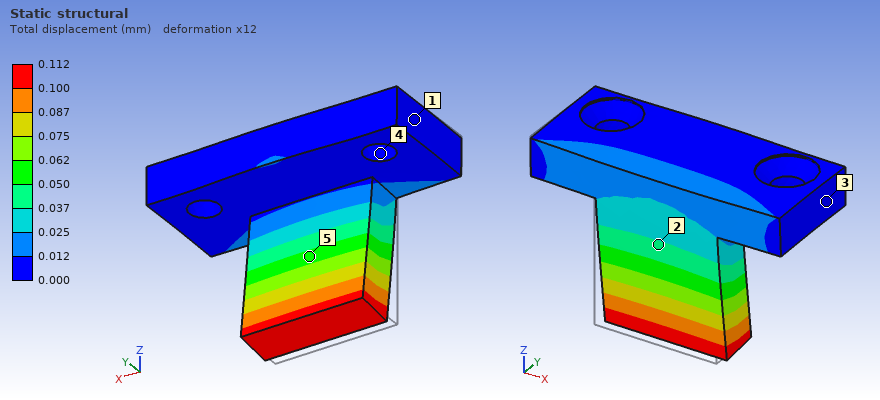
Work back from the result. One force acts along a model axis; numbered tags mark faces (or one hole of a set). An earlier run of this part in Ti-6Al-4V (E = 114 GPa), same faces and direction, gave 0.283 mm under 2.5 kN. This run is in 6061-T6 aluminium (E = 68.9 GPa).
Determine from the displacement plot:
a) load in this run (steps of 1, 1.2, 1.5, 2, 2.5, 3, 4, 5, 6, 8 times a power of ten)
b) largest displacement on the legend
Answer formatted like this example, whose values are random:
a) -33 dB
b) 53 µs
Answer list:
a) 600 N
b) 0.112 mm
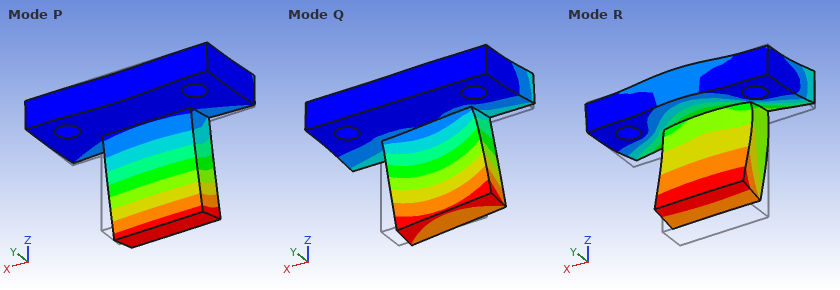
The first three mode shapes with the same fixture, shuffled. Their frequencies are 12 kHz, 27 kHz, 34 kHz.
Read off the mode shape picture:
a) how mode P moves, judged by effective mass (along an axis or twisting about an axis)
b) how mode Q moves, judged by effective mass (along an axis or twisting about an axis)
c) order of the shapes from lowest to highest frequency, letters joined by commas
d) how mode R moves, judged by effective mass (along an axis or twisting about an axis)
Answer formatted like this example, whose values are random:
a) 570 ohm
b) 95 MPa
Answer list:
a) along Y
b) along X
c) P, Q, R
d) along Z
